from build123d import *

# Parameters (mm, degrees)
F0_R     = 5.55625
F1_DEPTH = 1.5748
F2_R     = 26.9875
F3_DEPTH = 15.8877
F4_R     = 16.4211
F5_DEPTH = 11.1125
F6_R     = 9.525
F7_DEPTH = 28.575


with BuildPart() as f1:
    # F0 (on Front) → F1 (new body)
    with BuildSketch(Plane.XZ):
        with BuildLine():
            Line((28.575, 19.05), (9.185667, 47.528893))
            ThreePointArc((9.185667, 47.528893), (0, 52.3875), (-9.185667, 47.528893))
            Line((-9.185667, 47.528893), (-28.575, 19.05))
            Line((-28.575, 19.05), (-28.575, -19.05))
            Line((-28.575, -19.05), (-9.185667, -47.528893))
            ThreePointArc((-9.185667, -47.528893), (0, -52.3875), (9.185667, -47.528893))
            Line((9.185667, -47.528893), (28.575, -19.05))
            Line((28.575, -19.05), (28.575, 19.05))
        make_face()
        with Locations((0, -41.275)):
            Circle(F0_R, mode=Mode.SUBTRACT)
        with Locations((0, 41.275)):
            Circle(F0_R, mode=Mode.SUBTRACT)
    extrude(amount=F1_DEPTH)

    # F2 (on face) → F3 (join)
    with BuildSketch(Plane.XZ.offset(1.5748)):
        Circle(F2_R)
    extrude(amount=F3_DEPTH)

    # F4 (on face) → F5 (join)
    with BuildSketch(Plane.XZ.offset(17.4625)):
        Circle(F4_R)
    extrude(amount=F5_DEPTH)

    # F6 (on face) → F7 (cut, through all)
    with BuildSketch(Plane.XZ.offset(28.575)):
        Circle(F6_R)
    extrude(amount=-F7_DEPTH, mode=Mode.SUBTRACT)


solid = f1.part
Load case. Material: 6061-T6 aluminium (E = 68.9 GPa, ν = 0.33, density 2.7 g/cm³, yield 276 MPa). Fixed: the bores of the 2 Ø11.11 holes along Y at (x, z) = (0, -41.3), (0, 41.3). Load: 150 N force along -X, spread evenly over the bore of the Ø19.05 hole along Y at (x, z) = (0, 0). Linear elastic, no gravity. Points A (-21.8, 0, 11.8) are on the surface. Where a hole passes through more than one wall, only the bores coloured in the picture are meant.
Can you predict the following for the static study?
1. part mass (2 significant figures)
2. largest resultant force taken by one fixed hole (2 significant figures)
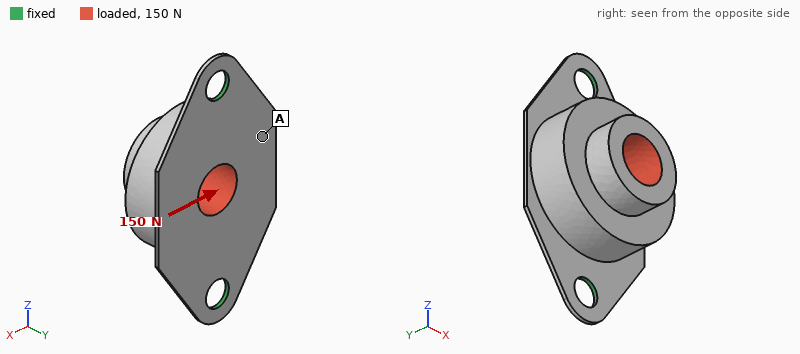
120 g
75 N
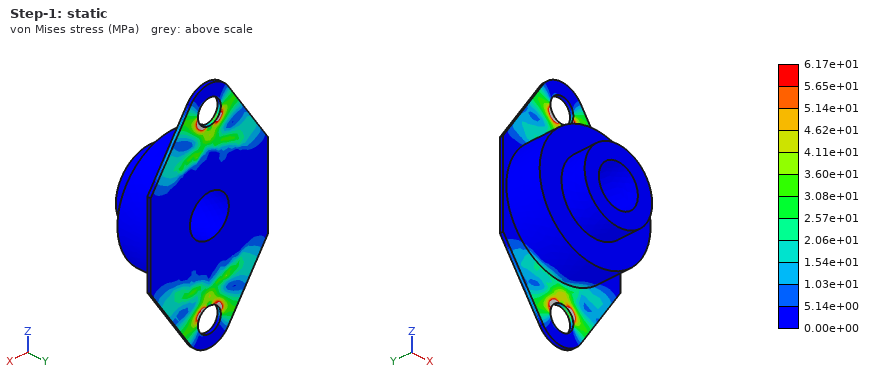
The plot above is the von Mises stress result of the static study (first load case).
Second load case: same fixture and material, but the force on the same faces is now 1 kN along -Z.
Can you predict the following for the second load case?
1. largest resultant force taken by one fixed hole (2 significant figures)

540 N
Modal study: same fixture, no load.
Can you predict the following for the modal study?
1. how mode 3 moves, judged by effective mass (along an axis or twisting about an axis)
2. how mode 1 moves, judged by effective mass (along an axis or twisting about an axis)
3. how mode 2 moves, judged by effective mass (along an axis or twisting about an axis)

along Z
along X
along Y
